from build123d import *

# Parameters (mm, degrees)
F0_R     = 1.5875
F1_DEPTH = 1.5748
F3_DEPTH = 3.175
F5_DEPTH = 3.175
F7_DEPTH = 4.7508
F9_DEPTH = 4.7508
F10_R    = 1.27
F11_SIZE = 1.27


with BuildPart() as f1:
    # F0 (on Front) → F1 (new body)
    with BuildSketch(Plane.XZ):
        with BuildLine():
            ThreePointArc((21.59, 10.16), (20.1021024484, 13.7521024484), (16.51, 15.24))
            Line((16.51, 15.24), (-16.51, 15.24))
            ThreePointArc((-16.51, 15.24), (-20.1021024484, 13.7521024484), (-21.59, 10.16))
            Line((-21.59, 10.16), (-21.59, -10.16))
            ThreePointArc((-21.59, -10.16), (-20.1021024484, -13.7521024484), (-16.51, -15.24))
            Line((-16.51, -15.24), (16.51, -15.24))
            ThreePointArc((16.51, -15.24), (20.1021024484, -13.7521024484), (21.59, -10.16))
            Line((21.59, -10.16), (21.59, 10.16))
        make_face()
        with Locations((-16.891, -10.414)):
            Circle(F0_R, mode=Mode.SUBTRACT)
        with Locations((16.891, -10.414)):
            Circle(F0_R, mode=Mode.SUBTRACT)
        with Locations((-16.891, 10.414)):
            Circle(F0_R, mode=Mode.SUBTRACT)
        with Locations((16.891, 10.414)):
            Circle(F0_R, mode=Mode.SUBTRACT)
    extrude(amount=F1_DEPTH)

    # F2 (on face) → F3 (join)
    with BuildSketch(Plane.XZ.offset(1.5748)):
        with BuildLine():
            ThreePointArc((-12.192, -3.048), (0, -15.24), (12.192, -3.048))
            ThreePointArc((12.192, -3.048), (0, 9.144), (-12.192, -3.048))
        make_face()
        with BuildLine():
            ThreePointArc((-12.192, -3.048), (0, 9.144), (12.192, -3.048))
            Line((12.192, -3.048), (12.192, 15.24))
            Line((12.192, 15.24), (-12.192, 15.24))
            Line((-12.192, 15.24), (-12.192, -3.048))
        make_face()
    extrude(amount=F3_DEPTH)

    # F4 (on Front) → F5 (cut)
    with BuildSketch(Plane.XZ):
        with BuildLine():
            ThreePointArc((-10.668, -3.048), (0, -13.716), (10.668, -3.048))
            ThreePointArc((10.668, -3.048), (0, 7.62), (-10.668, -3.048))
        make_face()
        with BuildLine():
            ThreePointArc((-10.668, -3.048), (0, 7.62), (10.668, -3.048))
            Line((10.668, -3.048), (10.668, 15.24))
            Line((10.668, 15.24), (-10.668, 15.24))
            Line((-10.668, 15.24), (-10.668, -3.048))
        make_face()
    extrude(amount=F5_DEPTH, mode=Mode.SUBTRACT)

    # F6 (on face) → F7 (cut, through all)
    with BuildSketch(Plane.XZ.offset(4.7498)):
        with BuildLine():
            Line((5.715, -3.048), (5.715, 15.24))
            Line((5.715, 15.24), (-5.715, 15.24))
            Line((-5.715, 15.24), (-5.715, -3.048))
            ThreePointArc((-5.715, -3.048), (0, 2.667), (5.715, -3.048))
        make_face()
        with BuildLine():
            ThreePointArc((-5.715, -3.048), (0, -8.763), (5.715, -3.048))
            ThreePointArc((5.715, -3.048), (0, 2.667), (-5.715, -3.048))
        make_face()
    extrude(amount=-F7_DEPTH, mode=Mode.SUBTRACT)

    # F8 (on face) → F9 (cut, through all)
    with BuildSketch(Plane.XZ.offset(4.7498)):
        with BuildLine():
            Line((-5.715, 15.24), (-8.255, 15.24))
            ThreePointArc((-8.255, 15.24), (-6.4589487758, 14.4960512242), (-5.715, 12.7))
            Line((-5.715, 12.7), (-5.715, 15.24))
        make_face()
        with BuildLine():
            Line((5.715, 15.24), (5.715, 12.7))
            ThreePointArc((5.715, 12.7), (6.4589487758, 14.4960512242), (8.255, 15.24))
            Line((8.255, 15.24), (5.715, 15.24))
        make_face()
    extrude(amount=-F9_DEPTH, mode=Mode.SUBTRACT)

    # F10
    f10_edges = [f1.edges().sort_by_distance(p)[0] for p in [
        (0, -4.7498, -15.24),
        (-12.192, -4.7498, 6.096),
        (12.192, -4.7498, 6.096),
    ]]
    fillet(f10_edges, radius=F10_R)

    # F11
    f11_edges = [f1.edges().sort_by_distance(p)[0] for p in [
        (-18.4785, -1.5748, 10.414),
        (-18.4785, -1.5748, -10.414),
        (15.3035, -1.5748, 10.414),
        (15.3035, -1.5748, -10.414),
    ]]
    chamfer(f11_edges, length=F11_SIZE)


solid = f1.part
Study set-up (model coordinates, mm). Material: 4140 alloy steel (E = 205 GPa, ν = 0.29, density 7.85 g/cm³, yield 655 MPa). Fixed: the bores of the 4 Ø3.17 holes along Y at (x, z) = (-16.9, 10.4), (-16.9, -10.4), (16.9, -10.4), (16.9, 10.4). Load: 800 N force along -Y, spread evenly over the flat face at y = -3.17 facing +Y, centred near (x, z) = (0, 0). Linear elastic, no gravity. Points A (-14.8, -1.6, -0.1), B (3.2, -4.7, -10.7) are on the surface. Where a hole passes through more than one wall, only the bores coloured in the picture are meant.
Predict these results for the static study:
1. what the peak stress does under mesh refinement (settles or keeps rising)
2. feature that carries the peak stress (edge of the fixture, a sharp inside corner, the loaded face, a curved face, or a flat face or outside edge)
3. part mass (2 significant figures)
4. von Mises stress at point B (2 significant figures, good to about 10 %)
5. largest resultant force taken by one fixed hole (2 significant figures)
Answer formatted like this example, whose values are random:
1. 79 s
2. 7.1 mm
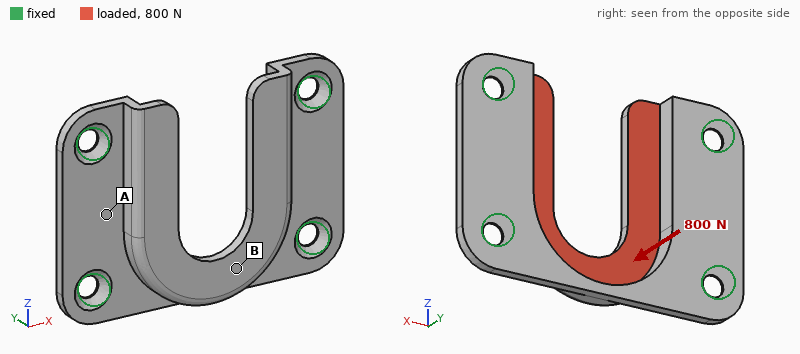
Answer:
1. keeps rising
2. edge of the fixture
3. 15 g
4. 110 MPa
5. 490 N
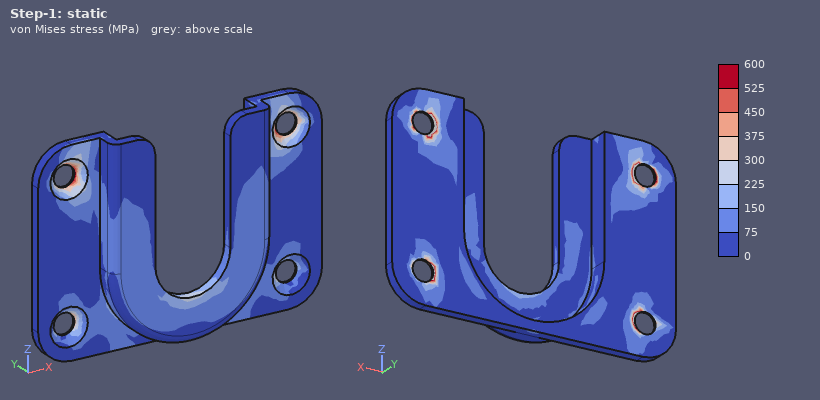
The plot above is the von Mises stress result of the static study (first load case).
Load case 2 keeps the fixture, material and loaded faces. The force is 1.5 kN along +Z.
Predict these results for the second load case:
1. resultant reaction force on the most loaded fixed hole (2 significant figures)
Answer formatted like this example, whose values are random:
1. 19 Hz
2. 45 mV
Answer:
1. 490 N
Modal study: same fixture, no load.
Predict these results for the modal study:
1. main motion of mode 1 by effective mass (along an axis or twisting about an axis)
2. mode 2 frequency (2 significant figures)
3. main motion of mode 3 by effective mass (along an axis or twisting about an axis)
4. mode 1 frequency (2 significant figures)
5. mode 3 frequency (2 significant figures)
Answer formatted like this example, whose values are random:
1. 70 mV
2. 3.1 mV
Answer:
1. along Y
2. 8400 Hz
3. along Y
4. 8000 Hz
5. 11 kHz
